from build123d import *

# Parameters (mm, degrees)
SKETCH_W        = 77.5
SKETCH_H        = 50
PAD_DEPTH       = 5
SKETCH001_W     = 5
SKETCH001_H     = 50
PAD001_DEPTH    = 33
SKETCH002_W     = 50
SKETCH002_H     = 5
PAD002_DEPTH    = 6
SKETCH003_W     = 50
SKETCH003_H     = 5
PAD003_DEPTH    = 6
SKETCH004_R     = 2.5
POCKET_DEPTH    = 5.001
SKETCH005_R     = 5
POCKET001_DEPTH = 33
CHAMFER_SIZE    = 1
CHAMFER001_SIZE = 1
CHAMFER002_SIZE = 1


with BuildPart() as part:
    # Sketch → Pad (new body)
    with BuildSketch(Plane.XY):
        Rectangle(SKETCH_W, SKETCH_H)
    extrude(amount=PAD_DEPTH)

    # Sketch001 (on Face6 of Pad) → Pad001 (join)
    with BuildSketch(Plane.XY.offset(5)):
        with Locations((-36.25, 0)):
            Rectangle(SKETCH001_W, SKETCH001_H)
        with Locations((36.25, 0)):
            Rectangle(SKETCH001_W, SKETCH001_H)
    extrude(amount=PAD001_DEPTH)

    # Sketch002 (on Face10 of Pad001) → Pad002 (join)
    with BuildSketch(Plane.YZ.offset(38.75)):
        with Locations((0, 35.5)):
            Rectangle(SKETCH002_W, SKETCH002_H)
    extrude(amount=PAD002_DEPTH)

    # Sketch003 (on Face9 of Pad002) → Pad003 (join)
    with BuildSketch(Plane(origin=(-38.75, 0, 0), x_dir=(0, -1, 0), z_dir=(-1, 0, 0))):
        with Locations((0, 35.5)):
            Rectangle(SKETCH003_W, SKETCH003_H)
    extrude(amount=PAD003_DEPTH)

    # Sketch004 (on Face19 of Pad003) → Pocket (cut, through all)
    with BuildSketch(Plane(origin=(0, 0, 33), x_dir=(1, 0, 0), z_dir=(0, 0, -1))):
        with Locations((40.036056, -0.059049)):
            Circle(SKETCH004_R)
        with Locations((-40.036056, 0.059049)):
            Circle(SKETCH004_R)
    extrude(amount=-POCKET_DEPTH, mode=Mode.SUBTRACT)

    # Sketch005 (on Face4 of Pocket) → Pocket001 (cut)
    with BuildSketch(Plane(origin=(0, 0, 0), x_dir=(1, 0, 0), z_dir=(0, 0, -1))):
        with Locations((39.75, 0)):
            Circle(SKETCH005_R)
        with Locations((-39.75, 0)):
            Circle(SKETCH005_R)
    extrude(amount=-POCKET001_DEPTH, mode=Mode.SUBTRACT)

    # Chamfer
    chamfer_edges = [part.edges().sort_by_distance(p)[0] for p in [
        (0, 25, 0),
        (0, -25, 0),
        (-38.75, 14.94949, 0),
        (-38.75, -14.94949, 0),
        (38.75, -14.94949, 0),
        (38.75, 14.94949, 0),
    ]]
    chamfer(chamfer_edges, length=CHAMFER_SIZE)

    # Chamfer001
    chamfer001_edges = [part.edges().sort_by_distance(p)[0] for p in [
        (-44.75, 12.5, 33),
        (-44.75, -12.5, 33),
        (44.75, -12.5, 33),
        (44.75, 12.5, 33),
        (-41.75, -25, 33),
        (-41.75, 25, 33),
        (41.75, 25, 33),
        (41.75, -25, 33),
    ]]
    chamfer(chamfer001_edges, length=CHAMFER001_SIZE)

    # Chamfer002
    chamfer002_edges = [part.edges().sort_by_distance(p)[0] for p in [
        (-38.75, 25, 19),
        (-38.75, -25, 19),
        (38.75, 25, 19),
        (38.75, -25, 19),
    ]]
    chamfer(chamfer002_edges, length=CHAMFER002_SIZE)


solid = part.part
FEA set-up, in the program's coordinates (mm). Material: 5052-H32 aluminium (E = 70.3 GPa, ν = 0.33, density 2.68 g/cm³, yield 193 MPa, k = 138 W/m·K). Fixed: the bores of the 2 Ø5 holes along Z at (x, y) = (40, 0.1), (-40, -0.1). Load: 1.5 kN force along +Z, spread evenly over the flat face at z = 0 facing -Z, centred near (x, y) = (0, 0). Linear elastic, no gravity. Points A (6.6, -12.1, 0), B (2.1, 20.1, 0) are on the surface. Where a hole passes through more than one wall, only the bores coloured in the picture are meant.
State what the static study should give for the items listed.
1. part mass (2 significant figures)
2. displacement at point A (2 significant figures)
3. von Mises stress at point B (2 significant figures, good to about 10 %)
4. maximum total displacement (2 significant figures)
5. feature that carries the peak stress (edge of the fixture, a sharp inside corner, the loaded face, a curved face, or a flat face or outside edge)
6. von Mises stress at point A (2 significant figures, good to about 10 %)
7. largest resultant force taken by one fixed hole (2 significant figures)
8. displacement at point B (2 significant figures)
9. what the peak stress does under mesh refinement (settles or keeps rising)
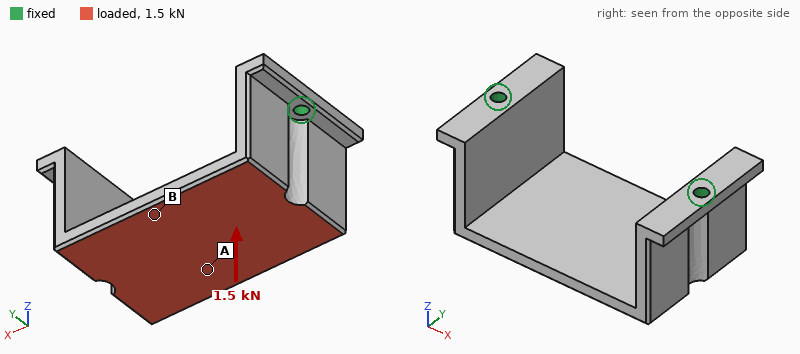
98 g
69 µm
30 MPa
79 µm
edge of the fixture
26 MPa
800 N
75 µm
keeps rising
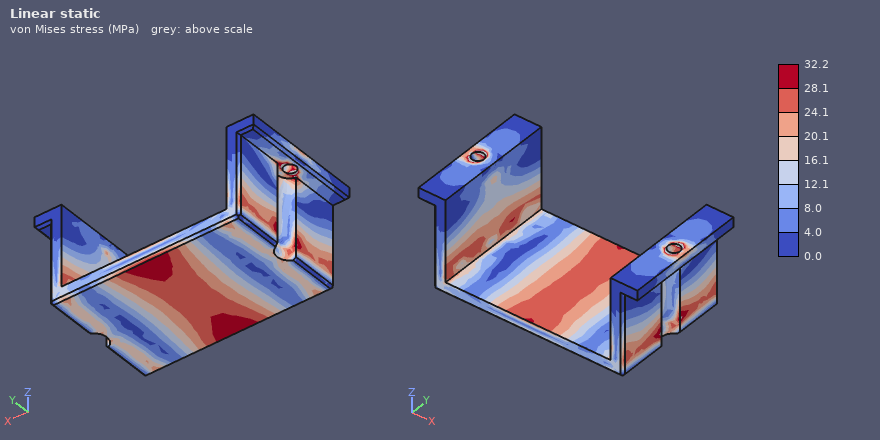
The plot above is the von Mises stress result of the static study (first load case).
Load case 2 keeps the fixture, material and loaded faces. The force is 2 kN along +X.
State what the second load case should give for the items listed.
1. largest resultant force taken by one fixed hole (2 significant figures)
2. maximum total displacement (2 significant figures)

1.1 kN
0.26 mm
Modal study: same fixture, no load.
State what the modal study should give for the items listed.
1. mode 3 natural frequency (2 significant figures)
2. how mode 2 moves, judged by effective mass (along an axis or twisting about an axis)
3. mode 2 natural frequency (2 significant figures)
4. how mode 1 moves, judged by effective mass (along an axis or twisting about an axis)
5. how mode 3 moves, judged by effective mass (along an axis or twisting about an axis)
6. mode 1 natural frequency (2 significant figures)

2500 Hz
along X
1800 Hz
along Y
twisting about Z
1700 Hz
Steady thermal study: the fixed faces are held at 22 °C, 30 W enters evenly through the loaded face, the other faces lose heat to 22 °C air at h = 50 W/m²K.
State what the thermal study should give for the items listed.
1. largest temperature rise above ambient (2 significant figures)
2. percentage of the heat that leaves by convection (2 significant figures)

23 K
30 %
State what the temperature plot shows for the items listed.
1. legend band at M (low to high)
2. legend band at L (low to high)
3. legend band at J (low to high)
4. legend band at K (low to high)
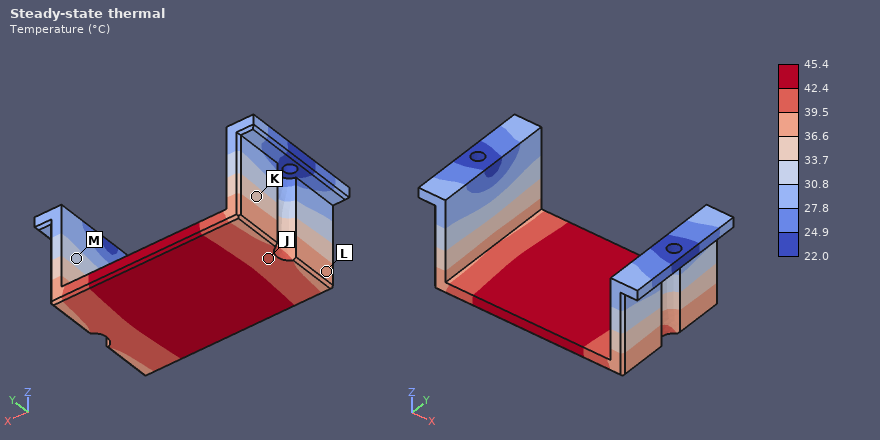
30.8 to 33.7 °C
36.6 to 39.5 °C
39.5 to 42.4 °C
33.7 to 36.6 °C
